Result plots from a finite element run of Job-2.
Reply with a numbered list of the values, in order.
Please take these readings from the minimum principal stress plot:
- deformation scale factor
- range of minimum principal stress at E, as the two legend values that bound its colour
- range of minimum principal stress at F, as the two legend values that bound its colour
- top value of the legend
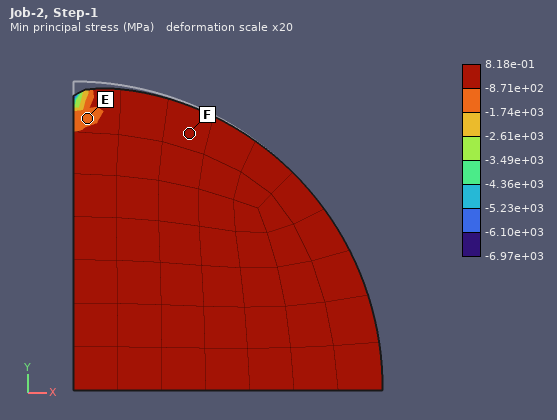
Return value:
1. 20
2. -1.74e+03 to -8.71e+02 MPa
3. -8.71e+02 to 8.18e-01 MPa
4. 8.18e-01 MPa
